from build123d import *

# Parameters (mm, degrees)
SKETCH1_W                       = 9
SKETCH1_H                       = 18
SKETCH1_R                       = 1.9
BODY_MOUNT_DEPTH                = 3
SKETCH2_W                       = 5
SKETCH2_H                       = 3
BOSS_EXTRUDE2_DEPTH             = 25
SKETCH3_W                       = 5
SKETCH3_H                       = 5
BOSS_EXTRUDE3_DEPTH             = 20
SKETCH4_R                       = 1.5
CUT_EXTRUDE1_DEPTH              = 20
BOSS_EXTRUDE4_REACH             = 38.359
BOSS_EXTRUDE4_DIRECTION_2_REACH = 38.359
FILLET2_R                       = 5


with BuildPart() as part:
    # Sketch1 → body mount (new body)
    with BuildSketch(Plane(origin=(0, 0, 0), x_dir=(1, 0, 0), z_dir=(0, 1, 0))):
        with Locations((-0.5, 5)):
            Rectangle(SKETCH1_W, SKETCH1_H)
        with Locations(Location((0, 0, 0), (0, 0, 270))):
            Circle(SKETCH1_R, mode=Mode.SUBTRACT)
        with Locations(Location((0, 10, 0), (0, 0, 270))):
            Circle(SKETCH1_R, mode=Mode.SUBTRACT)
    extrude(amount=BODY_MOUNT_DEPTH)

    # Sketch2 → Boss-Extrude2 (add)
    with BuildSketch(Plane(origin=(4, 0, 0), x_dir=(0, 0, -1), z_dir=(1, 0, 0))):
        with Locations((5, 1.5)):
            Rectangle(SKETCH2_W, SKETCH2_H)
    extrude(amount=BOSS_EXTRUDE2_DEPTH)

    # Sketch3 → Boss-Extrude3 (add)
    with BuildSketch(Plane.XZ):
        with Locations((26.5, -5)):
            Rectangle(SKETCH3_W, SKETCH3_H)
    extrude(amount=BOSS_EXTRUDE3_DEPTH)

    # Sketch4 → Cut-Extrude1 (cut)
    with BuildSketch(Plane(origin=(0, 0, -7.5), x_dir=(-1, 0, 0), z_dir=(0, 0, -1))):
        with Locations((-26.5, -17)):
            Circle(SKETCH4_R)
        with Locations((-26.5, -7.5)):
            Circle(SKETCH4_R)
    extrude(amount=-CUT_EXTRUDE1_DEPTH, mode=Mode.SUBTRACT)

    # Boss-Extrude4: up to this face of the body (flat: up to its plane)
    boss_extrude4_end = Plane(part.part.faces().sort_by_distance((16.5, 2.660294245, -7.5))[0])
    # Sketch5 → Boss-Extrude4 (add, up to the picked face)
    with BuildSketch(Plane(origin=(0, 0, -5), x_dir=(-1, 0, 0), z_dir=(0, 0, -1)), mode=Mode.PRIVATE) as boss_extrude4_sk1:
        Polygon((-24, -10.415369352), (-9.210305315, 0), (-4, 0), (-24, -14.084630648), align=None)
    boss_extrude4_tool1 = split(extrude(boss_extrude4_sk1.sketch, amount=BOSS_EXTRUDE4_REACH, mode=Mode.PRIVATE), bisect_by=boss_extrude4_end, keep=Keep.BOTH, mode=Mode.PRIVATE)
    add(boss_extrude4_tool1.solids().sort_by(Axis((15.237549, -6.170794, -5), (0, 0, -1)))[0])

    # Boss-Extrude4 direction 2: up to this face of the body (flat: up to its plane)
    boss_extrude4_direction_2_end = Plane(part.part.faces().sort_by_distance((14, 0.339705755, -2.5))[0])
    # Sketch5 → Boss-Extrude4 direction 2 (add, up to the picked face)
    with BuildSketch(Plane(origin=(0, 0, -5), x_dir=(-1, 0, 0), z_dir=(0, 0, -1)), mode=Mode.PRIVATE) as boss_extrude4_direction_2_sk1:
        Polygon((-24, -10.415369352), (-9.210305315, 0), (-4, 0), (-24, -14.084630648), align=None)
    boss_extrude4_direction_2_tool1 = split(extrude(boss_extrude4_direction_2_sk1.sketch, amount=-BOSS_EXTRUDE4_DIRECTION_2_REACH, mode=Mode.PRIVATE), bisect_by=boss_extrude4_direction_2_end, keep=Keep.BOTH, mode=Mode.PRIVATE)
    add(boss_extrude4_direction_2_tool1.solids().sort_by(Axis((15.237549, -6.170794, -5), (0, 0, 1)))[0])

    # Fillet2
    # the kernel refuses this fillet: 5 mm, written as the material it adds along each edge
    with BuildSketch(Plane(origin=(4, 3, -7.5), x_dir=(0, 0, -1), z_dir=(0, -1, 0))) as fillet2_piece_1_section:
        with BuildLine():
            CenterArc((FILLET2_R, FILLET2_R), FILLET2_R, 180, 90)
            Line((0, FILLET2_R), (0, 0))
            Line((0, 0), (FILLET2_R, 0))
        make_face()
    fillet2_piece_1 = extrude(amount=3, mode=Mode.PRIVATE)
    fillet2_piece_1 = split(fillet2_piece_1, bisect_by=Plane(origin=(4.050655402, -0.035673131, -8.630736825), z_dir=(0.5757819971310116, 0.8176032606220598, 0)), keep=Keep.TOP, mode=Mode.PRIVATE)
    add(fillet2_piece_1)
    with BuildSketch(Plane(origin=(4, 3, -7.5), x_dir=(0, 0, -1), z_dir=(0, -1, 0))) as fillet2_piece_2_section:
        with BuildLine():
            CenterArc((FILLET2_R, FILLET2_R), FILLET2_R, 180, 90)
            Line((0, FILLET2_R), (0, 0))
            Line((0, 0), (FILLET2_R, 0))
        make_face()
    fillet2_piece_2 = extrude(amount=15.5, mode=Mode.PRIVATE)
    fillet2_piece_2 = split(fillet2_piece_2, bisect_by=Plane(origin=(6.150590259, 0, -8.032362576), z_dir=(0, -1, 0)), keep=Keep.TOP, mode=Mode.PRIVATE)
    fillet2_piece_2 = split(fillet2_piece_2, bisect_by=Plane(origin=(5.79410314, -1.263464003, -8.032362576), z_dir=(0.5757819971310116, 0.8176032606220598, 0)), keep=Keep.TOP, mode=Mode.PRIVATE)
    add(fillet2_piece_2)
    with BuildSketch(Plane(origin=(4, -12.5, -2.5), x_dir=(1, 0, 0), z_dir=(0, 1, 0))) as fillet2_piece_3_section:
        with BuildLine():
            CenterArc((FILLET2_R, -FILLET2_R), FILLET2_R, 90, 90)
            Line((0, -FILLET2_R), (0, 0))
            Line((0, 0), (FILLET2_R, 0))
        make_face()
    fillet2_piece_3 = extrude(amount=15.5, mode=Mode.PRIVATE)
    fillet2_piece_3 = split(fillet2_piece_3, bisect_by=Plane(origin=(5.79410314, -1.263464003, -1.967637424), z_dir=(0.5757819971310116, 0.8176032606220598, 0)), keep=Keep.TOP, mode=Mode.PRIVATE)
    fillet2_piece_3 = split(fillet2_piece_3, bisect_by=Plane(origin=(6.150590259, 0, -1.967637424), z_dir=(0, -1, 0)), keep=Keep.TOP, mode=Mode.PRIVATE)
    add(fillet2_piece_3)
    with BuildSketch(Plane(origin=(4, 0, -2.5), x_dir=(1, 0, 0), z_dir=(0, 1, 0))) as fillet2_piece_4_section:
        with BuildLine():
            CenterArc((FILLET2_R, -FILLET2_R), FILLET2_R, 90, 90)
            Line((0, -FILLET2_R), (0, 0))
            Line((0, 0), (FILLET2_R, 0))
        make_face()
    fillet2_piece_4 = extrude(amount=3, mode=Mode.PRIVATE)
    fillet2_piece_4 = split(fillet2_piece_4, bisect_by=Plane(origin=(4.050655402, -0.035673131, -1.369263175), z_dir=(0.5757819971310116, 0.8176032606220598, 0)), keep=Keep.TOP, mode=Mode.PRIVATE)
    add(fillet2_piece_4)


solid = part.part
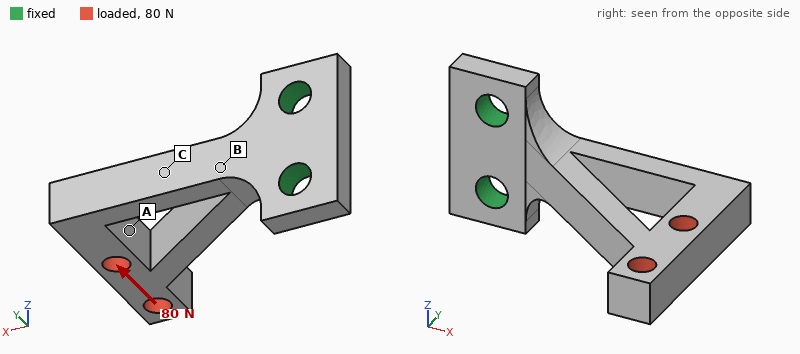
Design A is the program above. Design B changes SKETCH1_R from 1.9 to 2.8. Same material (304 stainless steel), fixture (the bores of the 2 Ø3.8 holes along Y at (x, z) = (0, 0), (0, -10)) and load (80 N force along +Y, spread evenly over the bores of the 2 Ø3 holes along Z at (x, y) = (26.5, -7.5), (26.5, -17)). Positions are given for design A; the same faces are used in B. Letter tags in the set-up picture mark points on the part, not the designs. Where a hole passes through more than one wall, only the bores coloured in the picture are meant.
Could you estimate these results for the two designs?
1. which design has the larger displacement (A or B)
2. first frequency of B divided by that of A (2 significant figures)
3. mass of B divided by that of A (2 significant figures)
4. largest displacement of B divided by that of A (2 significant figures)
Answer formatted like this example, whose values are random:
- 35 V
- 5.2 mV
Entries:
- A
- 1.1
- 0.95
- 0.90
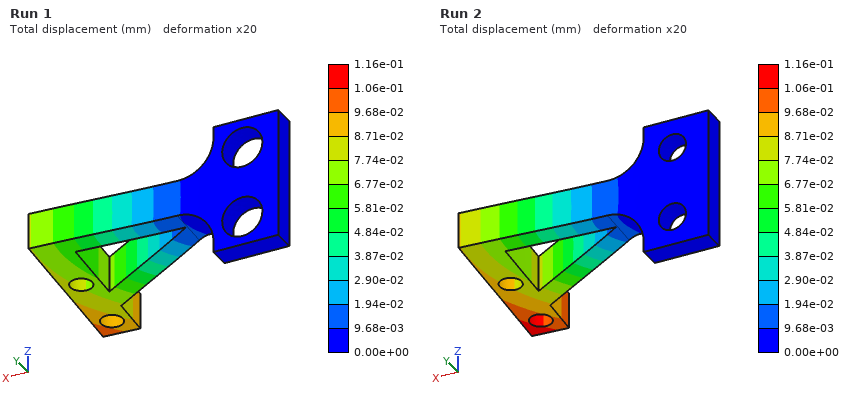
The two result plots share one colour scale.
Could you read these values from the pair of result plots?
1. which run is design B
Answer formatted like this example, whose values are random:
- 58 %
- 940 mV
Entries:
- Run 1
